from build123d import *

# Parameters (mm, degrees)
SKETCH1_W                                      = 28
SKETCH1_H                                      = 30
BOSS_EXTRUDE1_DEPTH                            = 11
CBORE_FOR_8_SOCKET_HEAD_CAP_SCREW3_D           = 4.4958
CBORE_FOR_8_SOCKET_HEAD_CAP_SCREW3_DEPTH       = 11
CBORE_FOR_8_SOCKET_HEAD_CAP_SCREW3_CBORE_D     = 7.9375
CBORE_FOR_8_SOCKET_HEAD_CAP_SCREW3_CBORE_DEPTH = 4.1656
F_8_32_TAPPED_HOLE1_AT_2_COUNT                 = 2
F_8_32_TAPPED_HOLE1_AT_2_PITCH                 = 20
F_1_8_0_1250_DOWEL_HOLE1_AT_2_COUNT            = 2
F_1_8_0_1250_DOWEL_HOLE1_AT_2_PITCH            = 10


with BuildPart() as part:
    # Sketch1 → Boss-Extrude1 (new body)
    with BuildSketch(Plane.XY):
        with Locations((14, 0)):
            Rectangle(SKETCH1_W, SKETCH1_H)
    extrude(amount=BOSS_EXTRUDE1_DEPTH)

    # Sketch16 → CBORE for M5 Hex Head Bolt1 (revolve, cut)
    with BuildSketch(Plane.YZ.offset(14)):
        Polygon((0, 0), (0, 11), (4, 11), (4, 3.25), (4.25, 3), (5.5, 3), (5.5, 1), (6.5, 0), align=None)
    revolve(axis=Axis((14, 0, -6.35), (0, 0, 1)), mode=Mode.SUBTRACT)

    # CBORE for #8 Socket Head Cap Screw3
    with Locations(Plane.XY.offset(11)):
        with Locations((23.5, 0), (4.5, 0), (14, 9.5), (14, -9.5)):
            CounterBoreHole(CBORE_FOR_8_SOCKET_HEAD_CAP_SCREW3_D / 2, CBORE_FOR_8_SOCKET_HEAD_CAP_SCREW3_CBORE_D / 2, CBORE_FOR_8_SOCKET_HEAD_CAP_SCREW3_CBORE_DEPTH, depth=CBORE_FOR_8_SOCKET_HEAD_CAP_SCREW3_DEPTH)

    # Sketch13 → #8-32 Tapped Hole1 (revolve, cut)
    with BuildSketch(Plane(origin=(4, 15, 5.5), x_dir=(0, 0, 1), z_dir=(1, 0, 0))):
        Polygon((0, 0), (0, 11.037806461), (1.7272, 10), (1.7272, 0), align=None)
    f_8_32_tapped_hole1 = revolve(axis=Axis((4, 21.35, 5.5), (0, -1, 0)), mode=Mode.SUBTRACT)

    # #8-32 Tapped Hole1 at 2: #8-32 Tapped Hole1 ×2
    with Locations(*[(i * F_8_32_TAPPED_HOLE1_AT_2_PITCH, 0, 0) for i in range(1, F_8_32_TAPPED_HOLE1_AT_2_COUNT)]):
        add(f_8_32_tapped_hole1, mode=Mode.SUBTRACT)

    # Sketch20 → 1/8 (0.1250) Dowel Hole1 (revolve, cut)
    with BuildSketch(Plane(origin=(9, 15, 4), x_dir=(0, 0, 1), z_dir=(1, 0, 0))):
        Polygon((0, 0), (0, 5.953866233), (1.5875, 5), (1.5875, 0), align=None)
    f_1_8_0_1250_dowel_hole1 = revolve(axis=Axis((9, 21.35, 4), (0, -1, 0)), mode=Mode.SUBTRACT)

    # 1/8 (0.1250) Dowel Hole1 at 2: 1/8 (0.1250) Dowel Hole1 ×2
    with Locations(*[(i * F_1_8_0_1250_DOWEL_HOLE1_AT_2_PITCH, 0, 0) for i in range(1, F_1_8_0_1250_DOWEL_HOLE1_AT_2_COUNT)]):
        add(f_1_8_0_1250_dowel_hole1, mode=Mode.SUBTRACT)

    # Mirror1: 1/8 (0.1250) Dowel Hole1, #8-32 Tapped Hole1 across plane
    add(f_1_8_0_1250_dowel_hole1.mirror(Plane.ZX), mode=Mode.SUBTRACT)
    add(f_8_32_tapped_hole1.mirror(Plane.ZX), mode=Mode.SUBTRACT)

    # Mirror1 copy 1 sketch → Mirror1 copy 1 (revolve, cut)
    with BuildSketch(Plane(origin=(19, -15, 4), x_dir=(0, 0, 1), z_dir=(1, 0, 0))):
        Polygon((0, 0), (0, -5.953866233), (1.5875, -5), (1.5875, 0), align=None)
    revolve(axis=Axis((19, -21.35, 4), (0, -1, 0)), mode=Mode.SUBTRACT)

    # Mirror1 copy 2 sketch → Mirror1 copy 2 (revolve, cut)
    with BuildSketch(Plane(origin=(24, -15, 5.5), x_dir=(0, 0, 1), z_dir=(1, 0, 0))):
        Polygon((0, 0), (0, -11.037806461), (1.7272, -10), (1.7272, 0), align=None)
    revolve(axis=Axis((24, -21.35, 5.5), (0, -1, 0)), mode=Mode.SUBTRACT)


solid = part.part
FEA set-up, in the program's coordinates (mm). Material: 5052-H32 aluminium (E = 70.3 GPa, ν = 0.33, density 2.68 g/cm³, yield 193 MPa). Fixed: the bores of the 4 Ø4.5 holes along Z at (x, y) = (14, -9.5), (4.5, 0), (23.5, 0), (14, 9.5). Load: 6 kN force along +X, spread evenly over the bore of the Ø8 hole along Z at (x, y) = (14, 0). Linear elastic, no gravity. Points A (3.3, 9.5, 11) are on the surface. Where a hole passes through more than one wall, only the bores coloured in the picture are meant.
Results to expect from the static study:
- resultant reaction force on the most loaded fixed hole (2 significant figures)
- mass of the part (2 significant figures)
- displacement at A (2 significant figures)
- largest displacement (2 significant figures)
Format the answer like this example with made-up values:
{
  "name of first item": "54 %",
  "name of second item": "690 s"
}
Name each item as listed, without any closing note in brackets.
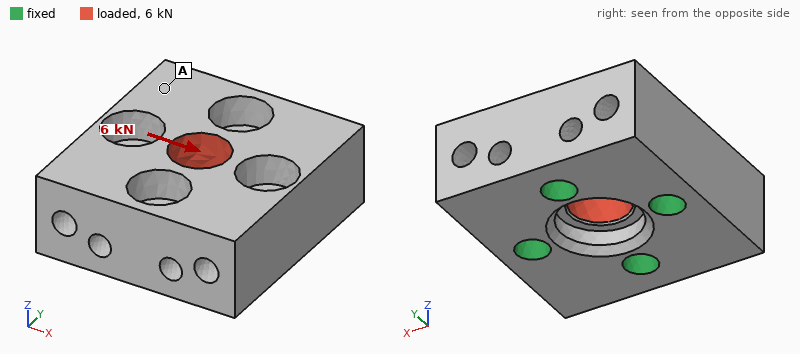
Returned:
{
  "resultant reaction force on the most loaded fixed hole": "1.9 kN",
  "mass of the part": "18 g",
  "displacement at A": "4.2 µm",
  "largest displacement": "11 µm"
}
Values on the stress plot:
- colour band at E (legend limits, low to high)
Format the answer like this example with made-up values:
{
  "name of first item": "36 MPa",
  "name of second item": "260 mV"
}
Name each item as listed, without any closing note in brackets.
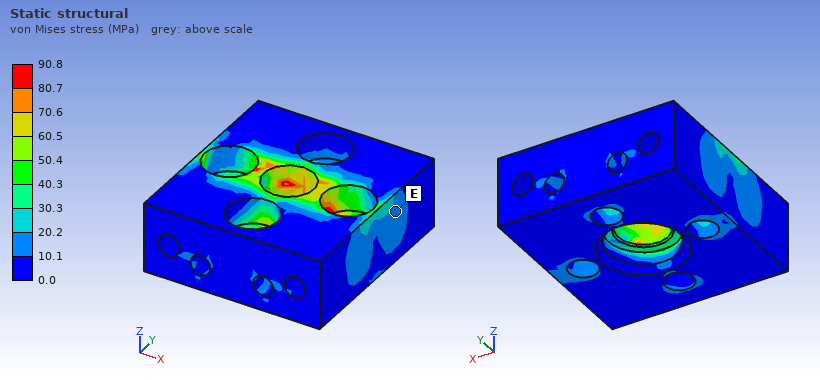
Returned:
{
  "colour band at E": "10.1 to 20.2 MPa"
}
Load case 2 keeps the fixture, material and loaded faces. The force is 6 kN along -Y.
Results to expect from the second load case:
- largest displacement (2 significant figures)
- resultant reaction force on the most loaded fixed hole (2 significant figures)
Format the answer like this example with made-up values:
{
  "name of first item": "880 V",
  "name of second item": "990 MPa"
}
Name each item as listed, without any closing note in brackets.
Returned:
{
  "largest displacement": "11 µm",
  "resultant reaction force on the most loaded fixed hole": "1.9 kN"
}
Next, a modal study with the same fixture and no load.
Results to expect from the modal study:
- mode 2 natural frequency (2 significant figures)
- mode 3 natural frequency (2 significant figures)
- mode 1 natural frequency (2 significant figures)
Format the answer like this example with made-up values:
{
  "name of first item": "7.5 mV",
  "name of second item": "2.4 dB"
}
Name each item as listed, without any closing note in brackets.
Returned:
{
  "mode 2 natural frequency": "38 kHz",
  "mode 3 natural frequency": "38 kHz",
  "mode 1 natural frequency": "35 kHz"
}
